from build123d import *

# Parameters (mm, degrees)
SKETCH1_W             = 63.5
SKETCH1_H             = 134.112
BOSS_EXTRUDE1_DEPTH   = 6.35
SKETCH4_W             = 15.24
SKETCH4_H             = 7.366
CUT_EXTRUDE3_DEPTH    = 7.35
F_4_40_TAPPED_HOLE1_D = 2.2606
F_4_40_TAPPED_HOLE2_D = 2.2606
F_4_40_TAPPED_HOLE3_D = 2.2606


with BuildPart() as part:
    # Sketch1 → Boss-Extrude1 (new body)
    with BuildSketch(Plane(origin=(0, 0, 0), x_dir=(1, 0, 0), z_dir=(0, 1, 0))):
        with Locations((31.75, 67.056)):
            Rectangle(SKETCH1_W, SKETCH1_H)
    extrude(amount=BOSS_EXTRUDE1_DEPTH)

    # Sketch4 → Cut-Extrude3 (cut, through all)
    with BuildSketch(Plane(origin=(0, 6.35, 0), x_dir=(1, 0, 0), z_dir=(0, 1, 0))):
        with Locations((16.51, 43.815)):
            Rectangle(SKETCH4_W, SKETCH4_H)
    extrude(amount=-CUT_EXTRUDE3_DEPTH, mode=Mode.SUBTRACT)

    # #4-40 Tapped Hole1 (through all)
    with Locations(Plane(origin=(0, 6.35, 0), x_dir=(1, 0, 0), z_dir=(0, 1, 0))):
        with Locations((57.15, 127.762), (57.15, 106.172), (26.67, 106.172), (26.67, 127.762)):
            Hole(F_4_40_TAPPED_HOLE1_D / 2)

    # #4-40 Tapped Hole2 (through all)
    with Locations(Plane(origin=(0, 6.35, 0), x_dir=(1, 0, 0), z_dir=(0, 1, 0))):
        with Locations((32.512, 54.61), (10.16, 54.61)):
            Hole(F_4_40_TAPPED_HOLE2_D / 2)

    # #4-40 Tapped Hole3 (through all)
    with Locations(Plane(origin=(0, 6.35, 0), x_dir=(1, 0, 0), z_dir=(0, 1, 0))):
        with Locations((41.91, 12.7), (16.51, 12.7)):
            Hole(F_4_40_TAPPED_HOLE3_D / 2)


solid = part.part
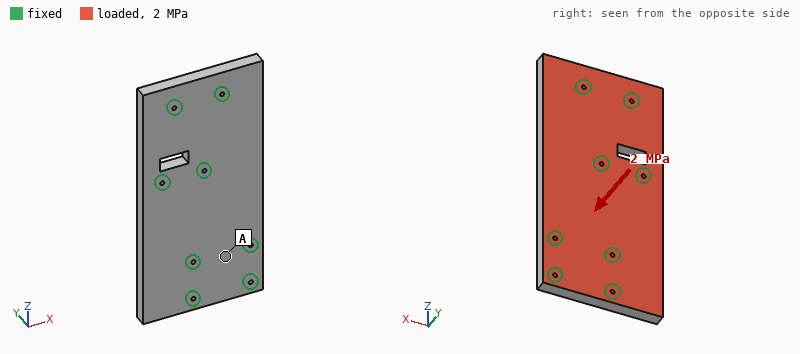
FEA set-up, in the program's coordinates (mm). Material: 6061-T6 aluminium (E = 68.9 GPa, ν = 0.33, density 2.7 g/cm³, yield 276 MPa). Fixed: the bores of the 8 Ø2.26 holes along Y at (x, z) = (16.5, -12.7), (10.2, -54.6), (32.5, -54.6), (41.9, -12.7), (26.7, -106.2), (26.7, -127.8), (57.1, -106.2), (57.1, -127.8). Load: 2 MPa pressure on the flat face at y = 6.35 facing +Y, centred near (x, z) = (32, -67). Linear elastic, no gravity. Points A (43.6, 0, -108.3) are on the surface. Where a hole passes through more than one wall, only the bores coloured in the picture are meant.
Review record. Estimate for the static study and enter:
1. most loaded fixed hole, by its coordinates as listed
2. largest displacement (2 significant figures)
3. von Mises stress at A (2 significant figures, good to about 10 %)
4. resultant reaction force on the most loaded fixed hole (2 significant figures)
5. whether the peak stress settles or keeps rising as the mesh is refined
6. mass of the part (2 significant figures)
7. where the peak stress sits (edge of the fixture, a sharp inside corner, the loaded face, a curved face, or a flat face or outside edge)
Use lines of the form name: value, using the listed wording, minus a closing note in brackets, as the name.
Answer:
most loaded fixed hole, by its coordinates as listed: (32.5, -54.6)
largest displacement: 0.16 mm
von Mises stress at A: 29 MPa
resultant reaction force on the most loaded fixed hole: 4.0 kN
whether the peak stress settles or keeps rising as the mesh is refined: keeps rising
mass of the part: 140 g
where the peak stress sits: edge of the fixture
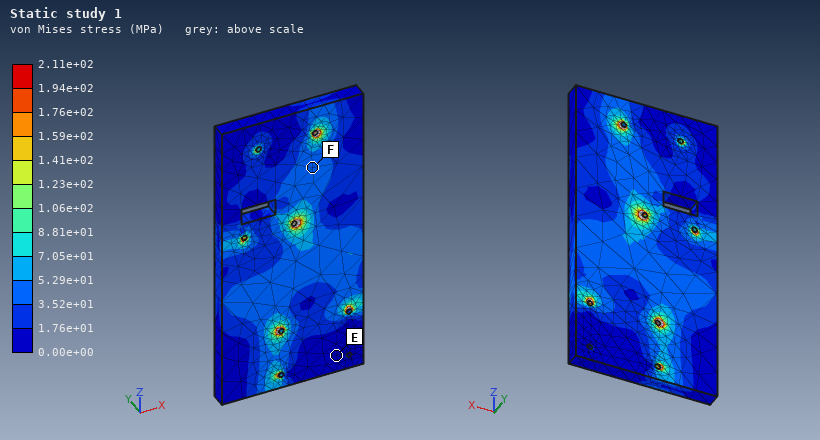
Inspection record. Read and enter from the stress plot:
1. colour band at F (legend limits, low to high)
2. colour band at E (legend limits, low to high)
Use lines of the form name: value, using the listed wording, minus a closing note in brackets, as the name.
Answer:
colour band at F: 3.52e+01 to 5.29e+01 MPa
colour band at E: 0.00e+00 to 1.76e+01 MPa
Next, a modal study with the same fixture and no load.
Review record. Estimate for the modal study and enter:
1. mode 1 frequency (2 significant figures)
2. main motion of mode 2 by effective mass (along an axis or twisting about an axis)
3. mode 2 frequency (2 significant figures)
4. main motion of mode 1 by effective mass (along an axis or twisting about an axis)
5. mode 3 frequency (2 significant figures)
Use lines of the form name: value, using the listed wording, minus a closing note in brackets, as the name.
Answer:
mode 1 frequency: 5600 Hz
main motion of mode 2 by effective mass: along Y
mode 2 frequency: 6400 Hz
main motion of mode 1 by effective mass: along Y
mode 3 frequency: 8400 Hz
